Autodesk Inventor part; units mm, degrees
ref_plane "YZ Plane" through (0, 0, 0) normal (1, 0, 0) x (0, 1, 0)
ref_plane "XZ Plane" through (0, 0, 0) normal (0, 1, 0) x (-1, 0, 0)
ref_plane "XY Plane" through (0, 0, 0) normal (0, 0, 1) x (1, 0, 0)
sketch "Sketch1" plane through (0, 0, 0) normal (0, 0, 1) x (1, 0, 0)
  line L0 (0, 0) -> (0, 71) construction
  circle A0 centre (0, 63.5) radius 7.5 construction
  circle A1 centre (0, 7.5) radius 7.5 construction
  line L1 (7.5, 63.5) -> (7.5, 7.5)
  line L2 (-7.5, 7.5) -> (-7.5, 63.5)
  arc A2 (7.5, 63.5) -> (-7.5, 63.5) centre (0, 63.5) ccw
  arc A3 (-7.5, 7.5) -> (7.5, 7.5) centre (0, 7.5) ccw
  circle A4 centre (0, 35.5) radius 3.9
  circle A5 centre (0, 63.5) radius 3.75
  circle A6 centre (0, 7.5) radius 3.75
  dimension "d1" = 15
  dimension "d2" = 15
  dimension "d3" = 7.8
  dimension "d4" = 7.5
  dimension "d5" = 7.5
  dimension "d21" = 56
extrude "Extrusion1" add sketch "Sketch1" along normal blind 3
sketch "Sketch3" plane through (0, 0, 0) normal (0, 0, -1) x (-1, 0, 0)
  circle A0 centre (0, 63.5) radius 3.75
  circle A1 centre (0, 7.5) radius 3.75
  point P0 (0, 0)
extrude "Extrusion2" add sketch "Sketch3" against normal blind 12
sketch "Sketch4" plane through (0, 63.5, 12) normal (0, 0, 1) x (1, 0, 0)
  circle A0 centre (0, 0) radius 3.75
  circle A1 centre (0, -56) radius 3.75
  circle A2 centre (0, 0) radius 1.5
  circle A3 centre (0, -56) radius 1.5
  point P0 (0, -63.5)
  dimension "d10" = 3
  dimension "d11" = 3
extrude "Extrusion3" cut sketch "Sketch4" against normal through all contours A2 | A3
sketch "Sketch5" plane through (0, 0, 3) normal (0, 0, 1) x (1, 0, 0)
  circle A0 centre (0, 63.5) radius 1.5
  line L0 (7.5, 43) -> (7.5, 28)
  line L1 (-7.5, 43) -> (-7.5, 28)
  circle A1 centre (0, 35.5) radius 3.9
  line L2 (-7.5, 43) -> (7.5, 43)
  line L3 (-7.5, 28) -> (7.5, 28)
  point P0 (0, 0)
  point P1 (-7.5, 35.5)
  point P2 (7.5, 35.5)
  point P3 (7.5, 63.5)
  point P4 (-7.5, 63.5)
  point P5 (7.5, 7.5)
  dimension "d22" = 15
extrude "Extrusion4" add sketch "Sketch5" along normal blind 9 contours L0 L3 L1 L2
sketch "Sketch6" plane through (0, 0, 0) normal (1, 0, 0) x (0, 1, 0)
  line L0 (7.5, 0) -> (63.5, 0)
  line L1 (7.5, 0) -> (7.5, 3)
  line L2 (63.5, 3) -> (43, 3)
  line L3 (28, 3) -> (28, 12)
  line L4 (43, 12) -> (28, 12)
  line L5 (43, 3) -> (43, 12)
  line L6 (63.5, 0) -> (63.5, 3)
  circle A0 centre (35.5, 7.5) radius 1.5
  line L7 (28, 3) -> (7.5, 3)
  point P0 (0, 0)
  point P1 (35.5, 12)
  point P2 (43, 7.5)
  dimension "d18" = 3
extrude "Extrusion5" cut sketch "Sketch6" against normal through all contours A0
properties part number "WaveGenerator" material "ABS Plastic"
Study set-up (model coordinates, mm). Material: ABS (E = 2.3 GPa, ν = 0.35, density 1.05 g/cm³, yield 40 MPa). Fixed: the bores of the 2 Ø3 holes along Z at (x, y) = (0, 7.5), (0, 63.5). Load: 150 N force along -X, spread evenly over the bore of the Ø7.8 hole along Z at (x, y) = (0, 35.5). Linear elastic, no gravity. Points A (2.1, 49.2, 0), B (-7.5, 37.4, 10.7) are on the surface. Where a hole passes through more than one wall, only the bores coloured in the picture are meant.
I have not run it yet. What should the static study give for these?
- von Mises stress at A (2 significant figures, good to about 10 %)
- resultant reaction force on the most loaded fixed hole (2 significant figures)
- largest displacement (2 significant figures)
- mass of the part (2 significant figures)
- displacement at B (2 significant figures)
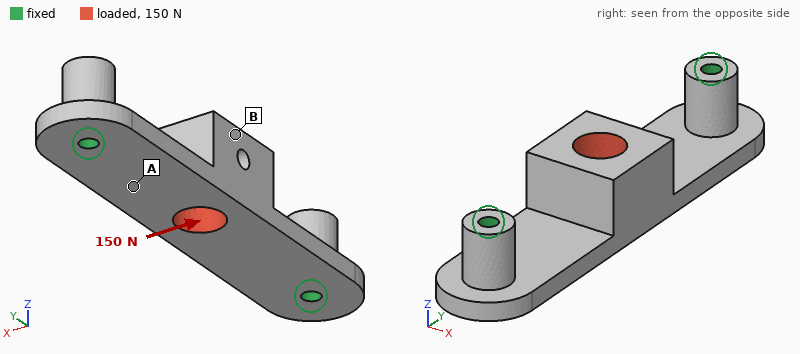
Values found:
8.7 MPa
75 N
0.87 mm
5.4 g
0.80 mm
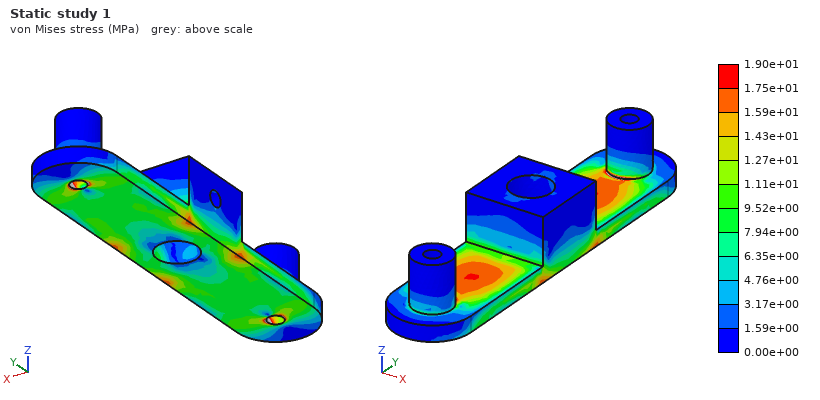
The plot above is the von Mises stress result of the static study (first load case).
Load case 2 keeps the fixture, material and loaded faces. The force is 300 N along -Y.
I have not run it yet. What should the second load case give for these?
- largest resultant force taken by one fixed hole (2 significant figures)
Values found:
150 N
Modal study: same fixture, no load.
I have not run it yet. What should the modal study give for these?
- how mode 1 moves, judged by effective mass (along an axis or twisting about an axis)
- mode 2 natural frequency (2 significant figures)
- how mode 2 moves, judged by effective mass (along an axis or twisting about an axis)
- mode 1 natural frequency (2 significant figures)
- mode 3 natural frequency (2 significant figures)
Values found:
along Z
1500 Hz
along X
1300 Hz
2900 Hz
